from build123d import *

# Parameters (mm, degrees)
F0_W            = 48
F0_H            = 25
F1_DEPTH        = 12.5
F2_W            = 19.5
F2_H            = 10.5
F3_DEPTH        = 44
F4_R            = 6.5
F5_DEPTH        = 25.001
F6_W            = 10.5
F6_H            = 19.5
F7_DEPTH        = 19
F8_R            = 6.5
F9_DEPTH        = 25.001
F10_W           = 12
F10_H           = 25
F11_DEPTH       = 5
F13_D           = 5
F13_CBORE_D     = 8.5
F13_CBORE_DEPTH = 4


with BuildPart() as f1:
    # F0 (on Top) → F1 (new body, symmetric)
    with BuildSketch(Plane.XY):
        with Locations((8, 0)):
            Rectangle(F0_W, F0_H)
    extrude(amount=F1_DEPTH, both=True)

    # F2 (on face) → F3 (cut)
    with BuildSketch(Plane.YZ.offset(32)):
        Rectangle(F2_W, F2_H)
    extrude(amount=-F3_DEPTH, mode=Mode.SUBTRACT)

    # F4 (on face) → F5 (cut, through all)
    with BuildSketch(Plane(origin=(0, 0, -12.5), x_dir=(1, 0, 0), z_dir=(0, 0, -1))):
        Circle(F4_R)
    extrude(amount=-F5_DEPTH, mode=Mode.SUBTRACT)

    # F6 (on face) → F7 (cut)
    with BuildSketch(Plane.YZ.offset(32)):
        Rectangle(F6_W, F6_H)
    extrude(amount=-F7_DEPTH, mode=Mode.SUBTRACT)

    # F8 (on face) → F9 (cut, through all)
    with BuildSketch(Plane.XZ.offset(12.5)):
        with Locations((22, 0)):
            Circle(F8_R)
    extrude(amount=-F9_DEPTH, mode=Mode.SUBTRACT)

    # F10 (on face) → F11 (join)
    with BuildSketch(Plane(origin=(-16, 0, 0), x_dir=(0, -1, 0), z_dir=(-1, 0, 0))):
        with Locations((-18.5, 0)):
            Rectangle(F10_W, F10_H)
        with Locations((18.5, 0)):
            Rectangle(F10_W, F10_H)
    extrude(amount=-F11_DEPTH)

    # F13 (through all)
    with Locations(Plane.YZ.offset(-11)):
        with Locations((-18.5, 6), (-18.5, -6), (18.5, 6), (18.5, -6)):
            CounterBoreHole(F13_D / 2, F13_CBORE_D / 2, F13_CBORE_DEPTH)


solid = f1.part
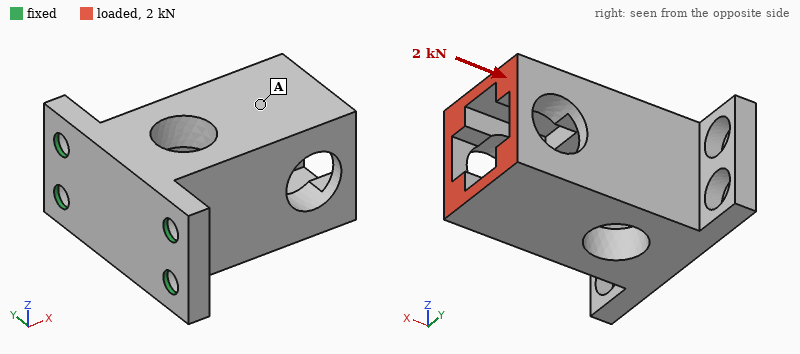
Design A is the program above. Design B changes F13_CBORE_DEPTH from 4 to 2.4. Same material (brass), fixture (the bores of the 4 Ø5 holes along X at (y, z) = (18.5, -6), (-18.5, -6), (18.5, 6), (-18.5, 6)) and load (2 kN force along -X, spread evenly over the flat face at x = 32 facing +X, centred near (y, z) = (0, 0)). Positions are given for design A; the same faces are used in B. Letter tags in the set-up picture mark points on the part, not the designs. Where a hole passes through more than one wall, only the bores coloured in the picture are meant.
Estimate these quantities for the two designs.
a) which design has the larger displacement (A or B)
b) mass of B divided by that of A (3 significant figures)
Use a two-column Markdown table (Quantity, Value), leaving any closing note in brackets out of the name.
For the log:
| Quantity | Value |
|---|---|
| which design has the larger displacement | A |
| mass of B divided by that of A | 1.01 |
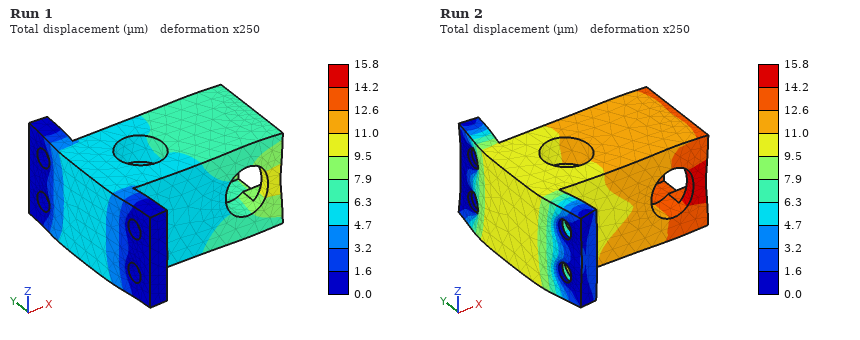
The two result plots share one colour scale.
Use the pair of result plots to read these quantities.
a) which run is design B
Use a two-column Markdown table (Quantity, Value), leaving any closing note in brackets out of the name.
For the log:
| Quantity | Value |
|---|---|
| which run is design B | Run 1 |
